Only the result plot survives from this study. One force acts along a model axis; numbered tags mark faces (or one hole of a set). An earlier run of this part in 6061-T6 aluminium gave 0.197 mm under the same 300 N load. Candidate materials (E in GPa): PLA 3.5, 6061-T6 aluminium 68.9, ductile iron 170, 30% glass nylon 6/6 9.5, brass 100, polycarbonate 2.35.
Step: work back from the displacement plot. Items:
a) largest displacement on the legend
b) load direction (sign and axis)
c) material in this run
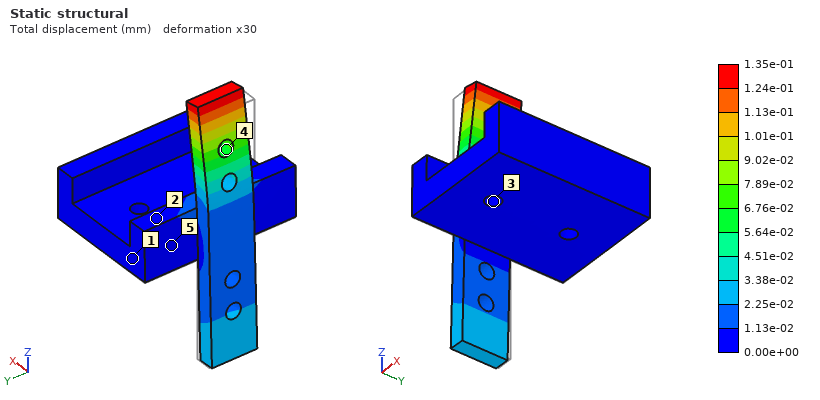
1.35e-01 mm
+X
brass
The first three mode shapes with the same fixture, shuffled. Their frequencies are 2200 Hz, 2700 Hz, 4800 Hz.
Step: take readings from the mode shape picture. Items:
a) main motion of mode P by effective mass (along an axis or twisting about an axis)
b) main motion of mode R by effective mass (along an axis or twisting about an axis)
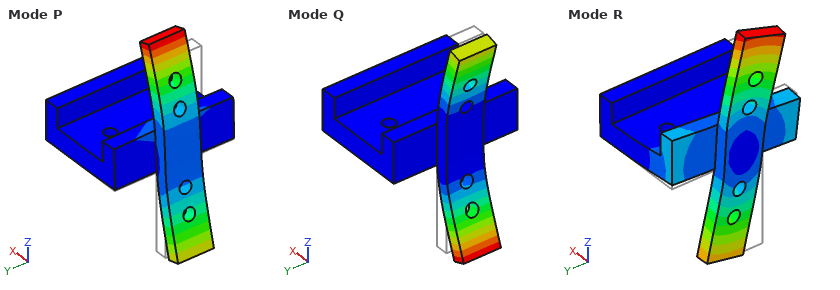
twisting about Y
twisting about X
